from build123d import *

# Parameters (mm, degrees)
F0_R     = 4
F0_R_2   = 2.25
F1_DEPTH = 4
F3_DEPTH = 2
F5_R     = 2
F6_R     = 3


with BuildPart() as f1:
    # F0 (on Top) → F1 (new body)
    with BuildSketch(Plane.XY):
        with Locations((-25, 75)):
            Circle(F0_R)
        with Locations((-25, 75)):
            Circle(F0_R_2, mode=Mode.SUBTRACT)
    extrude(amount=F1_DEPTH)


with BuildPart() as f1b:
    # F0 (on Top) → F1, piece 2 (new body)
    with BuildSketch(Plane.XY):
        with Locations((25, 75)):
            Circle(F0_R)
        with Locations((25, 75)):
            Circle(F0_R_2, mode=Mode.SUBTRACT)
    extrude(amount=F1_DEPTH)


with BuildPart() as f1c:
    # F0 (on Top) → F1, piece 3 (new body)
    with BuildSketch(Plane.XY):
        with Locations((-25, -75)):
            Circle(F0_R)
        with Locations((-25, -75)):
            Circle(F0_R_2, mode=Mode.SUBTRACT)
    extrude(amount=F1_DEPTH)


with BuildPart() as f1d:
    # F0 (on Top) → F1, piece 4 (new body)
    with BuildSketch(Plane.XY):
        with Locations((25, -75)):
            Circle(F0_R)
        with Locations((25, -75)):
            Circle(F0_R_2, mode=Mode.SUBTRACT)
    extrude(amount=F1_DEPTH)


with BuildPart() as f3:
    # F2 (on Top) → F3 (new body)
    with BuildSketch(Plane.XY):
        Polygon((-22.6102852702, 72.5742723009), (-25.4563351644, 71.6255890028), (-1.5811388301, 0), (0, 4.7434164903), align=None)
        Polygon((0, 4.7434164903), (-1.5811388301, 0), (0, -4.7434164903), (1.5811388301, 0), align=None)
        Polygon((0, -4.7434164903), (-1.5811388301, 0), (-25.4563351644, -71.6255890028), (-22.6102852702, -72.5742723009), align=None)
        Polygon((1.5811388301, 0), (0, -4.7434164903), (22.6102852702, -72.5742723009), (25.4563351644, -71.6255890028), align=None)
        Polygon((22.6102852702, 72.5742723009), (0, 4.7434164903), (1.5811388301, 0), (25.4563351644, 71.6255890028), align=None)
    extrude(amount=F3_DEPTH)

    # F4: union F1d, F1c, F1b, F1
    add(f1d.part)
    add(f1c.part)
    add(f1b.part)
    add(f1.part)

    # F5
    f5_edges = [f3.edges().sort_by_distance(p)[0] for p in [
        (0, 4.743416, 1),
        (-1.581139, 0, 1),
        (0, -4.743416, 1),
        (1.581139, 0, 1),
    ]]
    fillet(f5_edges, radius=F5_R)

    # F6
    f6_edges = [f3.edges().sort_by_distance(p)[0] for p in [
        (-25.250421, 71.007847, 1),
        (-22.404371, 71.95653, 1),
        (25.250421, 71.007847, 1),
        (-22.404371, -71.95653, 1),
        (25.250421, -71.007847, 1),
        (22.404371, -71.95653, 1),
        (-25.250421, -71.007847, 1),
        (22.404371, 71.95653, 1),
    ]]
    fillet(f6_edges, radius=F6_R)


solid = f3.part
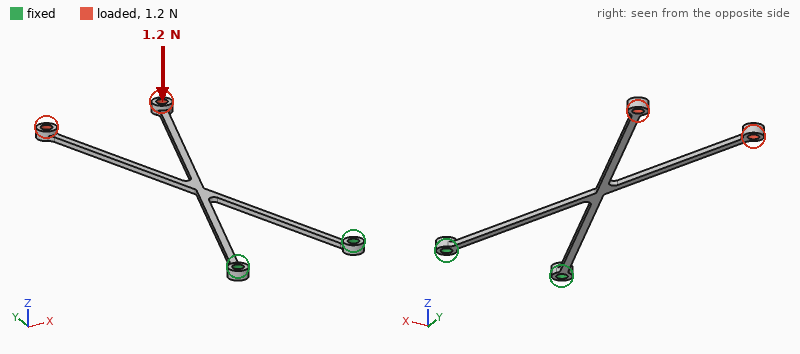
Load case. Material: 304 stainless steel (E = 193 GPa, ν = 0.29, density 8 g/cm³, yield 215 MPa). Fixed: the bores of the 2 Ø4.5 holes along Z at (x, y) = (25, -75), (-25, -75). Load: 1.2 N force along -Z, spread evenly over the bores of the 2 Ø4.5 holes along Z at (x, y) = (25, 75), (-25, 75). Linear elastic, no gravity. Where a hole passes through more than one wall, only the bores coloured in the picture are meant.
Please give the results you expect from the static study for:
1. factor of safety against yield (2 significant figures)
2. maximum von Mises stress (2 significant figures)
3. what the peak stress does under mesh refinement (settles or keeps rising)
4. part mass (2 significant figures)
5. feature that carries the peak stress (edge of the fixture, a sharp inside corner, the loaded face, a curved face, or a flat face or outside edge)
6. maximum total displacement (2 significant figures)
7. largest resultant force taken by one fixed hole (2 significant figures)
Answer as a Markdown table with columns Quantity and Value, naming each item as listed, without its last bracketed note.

| Quantity | Value |
|---|---|
| factor of safety against yield | 4.3 |
| maximum von Mises stress | 50 MPa |
| what the peak stress does under mesh refinement | settles |
| part mass | 19 g |
| feature that carries the peak stress | a curved face |
| maximum total displacement | 1.8 mm |
| largest resultant force taken by one fixed hole | 0.60 N |
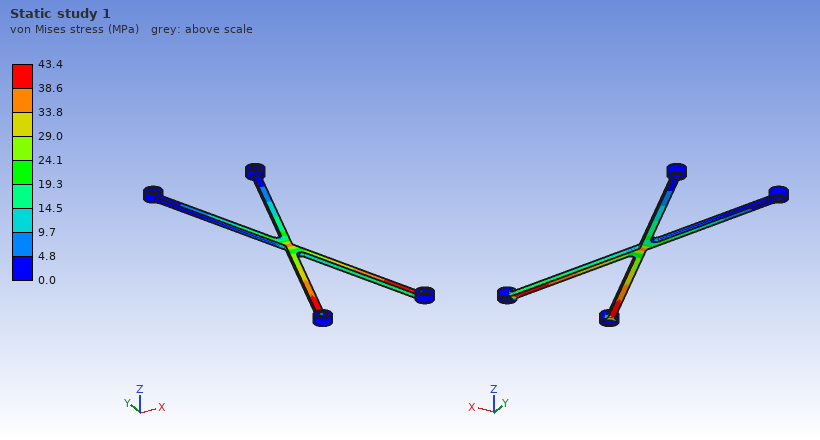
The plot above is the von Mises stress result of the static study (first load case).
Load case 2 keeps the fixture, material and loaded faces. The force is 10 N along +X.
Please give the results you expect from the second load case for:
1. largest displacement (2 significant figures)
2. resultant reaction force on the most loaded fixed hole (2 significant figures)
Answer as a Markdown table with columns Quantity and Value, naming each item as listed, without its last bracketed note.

| Quantity | Value |
|---|---|
| largest displacement | 1.4 mm |
| resultant reaction force on the most loaded fixed hole | 38 N |
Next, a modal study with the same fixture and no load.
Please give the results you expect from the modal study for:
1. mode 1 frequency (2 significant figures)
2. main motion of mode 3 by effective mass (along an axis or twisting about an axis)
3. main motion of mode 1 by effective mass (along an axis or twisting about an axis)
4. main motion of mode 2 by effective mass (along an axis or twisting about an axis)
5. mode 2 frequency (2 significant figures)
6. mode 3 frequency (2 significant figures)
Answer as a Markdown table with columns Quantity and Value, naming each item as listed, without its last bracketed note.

| Quantity | Value |
|---|---|
| mode 1 frequency | 56 Hz |
| main motion of mode 3 by effective mass | along X |
| main motion of mode 1 by effective mass | along Z |
| main motion of mode 2 by effective mass | twisting about Y |
| mode 2 frequency | 180 Hz |
| mode 3 frequency | 210 Hz |
